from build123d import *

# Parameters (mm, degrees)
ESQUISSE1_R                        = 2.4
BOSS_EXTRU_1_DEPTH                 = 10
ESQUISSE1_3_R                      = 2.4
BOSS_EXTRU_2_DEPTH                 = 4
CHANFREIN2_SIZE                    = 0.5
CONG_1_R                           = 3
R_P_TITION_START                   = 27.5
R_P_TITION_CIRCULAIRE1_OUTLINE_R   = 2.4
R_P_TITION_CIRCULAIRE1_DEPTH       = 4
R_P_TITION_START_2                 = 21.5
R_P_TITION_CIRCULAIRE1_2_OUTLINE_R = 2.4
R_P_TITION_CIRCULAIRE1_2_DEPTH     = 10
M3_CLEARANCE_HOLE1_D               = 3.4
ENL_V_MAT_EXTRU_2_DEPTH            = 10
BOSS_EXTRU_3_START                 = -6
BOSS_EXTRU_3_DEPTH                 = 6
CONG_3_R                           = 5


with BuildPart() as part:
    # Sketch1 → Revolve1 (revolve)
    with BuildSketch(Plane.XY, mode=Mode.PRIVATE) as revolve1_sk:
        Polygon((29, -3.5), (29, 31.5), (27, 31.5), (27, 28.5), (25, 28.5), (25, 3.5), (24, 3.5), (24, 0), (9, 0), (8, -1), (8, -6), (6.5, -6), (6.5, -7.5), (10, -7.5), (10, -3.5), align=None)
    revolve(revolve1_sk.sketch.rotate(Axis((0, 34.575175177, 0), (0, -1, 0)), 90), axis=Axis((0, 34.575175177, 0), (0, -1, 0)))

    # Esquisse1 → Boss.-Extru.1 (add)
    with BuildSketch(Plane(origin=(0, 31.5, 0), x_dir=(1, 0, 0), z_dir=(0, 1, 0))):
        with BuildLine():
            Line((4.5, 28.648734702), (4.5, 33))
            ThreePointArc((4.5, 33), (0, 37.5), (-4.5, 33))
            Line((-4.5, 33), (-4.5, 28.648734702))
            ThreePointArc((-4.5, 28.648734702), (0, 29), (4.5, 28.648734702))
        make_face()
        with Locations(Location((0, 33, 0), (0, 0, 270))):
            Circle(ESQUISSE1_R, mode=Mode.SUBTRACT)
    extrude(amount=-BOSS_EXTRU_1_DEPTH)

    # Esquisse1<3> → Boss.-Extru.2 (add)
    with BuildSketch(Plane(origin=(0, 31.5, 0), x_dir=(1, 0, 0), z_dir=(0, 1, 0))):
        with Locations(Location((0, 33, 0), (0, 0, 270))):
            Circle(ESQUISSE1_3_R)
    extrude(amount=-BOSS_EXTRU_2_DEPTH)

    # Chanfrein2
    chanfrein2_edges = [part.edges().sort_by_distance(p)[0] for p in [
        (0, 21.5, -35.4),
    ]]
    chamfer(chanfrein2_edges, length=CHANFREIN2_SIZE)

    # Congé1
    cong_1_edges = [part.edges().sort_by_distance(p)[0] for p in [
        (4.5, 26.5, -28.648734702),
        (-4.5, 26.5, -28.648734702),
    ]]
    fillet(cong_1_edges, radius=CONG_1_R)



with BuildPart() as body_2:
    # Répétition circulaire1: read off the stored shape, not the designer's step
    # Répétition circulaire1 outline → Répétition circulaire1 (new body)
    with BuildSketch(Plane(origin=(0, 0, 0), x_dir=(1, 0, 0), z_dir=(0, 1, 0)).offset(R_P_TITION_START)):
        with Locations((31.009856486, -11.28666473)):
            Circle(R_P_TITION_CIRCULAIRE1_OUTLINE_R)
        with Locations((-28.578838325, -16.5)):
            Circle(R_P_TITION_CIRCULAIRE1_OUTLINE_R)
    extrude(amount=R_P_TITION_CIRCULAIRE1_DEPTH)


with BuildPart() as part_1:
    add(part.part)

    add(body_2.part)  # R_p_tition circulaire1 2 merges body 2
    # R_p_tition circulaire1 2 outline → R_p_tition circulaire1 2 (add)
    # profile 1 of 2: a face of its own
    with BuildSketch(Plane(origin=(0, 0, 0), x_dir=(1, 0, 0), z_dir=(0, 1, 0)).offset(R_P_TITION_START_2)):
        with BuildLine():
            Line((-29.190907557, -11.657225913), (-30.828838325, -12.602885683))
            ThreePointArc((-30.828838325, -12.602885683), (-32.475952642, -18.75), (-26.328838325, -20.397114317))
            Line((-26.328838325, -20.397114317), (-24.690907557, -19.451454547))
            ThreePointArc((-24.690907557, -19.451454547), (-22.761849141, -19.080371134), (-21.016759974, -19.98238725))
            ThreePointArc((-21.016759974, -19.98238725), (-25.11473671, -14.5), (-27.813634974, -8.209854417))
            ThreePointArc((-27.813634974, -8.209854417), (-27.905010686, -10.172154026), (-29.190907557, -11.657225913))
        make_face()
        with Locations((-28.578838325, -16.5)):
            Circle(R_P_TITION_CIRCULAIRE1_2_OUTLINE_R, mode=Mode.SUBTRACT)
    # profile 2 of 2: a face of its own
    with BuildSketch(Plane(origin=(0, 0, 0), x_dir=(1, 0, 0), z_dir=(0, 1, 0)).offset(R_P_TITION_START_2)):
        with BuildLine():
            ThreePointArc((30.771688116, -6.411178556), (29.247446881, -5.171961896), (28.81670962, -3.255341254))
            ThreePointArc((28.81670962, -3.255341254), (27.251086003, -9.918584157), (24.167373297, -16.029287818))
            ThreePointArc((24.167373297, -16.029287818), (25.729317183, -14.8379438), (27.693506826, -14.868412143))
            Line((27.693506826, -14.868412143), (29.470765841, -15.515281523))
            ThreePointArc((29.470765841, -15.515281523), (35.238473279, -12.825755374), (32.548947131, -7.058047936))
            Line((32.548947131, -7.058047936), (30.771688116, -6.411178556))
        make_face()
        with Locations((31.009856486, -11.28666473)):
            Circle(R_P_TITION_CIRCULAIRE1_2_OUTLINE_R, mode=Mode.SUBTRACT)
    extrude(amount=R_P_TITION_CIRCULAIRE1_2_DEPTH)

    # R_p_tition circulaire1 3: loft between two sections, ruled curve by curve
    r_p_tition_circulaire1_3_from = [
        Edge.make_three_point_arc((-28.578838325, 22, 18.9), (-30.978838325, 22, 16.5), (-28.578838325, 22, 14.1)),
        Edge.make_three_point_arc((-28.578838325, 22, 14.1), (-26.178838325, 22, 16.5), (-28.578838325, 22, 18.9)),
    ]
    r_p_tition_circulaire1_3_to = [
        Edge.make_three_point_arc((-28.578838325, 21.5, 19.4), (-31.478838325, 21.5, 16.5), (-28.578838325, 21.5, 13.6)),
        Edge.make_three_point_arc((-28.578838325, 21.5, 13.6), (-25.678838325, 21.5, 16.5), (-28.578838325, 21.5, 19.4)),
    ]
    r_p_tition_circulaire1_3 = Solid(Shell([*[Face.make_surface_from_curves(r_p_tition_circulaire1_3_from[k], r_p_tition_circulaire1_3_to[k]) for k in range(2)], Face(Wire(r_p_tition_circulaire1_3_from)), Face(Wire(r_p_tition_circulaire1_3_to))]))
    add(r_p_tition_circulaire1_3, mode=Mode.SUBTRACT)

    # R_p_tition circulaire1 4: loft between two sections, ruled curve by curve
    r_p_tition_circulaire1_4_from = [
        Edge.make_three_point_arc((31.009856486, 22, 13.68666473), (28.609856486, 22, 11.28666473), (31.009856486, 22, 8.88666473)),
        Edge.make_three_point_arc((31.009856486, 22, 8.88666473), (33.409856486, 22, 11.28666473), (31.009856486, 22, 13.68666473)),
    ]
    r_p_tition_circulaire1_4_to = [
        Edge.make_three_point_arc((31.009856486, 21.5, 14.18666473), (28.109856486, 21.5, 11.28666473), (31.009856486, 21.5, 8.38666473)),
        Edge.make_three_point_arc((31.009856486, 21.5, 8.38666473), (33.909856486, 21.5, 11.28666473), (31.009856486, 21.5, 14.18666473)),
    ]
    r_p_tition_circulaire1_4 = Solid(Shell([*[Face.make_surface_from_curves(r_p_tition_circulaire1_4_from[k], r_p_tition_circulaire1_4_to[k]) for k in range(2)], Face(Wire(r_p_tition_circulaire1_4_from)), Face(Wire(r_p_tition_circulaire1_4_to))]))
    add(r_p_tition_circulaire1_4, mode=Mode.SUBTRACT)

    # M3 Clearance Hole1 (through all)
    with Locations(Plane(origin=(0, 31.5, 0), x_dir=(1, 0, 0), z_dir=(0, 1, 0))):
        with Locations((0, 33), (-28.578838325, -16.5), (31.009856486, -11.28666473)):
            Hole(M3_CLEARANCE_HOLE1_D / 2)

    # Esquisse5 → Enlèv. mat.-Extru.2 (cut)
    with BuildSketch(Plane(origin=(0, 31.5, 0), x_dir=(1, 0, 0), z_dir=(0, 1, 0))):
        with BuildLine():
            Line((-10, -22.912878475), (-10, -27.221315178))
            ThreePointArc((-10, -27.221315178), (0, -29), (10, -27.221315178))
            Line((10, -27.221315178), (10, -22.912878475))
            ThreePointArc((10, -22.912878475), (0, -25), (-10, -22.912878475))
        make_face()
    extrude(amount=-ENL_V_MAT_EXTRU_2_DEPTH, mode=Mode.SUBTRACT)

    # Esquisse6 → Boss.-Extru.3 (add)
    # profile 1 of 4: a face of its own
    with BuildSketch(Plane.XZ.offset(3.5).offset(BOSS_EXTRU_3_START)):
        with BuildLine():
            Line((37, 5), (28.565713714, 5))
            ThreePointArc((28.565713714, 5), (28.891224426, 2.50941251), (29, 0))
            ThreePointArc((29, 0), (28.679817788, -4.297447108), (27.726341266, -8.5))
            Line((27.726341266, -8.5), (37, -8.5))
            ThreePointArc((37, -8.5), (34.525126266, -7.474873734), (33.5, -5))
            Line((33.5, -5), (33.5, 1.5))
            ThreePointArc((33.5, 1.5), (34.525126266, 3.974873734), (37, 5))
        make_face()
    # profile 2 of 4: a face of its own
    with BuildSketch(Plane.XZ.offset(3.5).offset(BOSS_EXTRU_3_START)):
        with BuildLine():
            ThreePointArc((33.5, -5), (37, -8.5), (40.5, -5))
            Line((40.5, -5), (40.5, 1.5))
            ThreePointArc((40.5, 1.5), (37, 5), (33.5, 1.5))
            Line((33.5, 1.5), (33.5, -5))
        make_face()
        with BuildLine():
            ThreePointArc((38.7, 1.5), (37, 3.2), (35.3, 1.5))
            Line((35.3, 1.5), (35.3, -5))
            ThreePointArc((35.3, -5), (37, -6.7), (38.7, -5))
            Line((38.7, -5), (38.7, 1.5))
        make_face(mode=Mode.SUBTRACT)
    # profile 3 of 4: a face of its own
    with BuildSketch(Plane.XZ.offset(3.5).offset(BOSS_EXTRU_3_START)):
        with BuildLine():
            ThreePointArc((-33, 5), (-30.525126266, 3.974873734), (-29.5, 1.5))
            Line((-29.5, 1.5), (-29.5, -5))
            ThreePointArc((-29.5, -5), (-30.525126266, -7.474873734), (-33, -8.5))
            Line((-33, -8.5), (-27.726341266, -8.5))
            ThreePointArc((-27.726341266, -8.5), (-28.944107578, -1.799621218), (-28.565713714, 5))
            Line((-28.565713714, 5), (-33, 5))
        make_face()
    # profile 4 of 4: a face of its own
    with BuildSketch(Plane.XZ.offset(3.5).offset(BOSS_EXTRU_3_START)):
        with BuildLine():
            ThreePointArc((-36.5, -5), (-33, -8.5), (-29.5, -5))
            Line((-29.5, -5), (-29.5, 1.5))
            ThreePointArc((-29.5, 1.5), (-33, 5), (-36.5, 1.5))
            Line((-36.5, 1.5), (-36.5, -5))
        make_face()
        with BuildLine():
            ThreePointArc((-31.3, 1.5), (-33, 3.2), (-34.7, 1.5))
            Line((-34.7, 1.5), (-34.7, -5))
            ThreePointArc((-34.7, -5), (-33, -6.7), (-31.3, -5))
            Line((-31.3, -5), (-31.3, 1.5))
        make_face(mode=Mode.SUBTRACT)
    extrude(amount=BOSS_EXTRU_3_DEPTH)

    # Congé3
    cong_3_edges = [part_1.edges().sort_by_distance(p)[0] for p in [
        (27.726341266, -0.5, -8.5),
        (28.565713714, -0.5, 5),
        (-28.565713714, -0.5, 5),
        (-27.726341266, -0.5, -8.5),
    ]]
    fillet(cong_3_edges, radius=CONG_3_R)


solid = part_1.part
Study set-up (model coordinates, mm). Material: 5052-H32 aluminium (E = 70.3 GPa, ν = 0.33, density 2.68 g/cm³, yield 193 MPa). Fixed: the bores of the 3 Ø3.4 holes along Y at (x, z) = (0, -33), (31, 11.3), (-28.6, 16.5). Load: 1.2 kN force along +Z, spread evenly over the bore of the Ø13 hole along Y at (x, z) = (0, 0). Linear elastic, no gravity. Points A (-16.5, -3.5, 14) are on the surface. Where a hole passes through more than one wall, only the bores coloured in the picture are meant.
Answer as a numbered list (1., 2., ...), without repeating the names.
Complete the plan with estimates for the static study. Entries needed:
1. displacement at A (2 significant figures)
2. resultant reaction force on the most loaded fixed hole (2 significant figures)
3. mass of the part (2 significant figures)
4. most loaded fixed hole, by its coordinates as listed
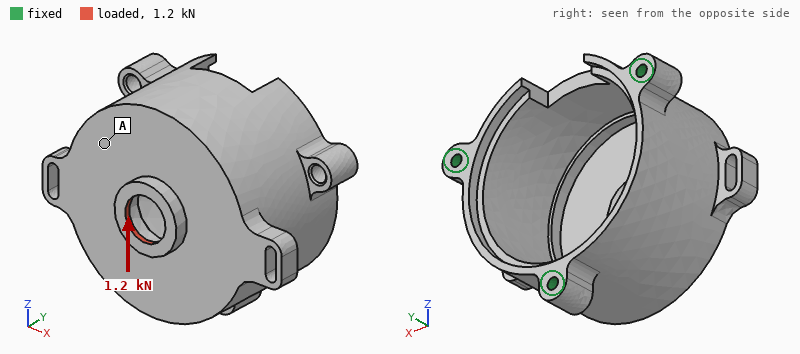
1. 16 µm
2. 1.1 kN
3. 86 g
4. (0, -33)
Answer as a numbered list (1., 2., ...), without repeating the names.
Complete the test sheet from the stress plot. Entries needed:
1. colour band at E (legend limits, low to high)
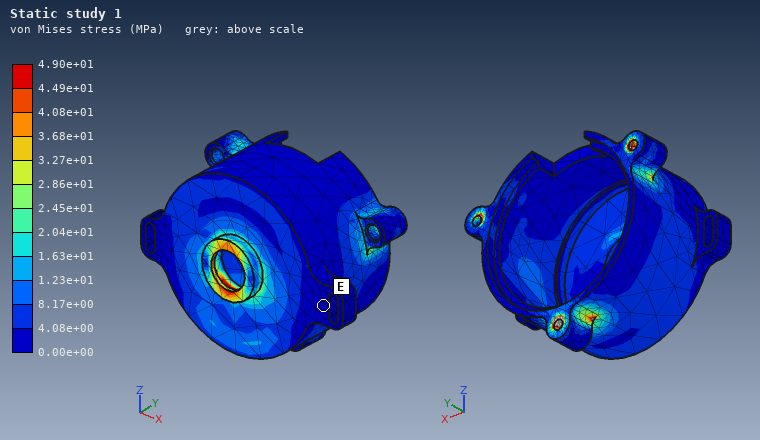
1. 0.00e+00 to 4.08e+00 MPa
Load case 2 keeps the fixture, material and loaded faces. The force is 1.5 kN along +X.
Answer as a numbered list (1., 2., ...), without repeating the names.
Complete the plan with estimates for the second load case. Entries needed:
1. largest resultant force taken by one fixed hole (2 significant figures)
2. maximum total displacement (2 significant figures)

1. 1.1 kN
2. 32 µm
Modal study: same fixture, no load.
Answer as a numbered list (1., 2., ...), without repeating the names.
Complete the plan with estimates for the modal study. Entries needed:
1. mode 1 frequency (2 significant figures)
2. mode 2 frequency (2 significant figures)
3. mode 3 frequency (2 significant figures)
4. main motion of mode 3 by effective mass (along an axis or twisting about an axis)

1. 6300 Hz
2. 6700 Hz
3. 9300 Hz
4. along Y
